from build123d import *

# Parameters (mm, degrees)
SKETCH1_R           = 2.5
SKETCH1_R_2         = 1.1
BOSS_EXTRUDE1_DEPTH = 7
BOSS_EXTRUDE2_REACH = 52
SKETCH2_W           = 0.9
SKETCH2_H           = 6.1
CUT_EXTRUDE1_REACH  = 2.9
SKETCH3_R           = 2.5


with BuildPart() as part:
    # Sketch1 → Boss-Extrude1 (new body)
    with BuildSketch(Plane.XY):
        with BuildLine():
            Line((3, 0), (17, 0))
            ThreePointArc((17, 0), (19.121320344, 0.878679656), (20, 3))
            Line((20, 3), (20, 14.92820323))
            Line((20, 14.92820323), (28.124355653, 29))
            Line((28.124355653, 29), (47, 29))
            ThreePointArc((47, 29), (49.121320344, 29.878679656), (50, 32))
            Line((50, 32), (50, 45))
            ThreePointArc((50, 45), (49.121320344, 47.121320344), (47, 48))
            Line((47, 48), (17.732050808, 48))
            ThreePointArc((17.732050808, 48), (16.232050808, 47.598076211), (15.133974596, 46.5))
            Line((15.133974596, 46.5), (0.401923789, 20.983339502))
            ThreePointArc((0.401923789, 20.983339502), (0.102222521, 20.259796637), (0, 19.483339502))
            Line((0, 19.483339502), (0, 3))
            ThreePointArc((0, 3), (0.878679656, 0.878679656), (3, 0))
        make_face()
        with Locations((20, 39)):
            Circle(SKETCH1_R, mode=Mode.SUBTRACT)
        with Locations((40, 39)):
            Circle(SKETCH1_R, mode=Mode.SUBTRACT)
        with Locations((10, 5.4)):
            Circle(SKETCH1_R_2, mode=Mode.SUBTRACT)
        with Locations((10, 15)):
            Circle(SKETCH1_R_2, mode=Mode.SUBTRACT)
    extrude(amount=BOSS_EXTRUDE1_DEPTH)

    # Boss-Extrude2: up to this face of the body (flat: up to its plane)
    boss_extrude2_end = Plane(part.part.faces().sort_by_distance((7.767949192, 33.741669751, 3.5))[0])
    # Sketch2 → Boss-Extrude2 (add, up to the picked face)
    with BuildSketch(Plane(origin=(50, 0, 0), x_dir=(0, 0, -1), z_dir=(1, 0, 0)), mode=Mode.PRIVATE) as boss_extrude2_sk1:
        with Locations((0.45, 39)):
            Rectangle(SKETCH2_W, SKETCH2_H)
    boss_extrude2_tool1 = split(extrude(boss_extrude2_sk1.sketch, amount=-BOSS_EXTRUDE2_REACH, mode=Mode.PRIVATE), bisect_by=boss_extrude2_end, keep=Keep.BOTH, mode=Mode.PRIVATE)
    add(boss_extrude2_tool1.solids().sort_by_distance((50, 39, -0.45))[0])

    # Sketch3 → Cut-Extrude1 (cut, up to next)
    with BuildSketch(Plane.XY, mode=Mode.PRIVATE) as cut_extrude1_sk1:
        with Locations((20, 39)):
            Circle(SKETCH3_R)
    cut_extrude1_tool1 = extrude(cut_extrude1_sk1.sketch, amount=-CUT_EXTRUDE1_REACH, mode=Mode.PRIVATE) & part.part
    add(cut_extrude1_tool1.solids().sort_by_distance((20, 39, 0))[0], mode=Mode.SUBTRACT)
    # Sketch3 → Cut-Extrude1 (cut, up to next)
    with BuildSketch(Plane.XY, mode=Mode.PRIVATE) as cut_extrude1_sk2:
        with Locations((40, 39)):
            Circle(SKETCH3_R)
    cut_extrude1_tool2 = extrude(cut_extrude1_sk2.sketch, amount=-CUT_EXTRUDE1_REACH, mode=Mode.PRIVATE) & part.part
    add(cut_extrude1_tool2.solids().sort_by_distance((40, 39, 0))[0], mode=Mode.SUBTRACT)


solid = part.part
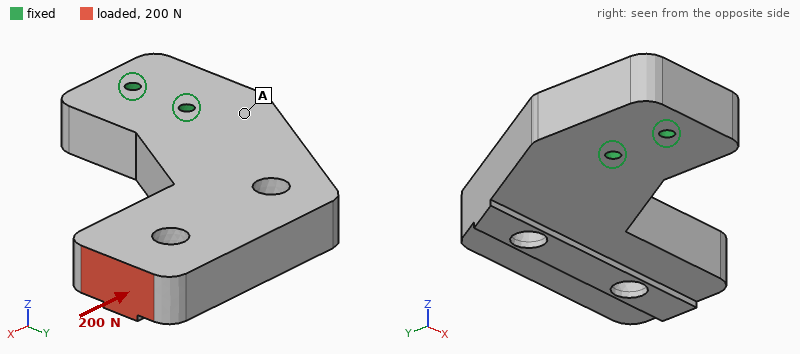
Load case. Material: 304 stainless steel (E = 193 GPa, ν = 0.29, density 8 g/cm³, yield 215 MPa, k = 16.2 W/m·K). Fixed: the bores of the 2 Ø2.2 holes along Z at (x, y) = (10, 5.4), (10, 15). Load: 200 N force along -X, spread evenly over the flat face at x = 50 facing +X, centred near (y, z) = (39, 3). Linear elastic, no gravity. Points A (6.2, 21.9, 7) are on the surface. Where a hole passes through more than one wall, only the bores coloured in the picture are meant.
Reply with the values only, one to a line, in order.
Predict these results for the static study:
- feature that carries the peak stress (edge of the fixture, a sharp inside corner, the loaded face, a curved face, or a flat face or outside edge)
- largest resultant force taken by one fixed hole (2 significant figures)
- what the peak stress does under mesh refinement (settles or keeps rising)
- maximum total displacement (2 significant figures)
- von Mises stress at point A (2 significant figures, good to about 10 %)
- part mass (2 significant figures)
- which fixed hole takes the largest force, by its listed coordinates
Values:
edge of the fixture
600 N
keeps rising
7.6 µm
4.7 MPa
75 g
(10, 15)
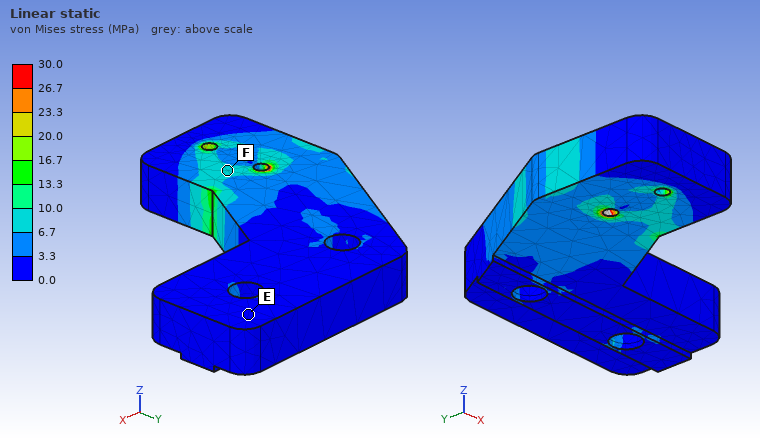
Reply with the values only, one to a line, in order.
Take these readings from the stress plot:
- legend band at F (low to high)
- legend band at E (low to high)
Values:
6.7 to 10.0 MPa
0.0 to 3.3 MPa
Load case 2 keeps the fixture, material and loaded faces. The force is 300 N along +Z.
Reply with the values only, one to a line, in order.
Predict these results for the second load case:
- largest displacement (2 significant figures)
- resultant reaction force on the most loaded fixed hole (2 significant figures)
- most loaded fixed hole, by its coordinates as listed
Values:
0.13 mm
580 N
(10, 15)
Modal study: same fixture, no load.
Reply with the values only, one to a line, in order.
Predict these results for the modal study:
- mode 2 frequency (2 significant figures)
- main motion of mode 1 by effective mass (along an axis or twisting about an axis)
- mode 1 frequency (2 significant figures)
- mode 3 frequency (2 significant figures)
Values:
4100 Hz
along Z
2100 Hz
6100 Hz
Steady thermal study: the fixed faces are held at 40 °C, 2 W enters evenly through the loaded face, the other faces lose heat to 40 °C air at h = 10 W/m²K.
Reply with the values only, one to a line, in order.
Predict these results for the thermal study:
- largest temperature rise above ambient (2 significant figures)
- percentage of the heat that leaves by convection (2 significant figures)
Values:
42 K
31 %
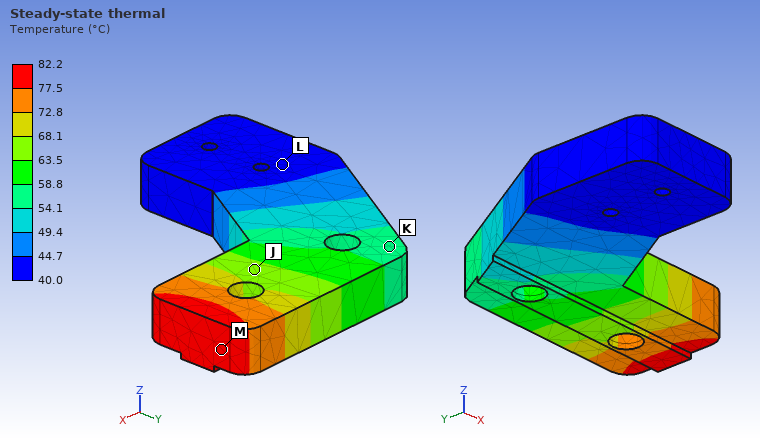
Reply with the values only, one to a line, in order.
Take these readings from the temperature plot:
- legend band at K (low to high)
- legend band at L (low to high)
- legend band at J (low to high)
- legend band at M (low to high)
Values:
54.1 to 58.8 °C
40.0 to 44.7 °C
63.5 to 68.1 °C
77.5 to 82.2 °C
